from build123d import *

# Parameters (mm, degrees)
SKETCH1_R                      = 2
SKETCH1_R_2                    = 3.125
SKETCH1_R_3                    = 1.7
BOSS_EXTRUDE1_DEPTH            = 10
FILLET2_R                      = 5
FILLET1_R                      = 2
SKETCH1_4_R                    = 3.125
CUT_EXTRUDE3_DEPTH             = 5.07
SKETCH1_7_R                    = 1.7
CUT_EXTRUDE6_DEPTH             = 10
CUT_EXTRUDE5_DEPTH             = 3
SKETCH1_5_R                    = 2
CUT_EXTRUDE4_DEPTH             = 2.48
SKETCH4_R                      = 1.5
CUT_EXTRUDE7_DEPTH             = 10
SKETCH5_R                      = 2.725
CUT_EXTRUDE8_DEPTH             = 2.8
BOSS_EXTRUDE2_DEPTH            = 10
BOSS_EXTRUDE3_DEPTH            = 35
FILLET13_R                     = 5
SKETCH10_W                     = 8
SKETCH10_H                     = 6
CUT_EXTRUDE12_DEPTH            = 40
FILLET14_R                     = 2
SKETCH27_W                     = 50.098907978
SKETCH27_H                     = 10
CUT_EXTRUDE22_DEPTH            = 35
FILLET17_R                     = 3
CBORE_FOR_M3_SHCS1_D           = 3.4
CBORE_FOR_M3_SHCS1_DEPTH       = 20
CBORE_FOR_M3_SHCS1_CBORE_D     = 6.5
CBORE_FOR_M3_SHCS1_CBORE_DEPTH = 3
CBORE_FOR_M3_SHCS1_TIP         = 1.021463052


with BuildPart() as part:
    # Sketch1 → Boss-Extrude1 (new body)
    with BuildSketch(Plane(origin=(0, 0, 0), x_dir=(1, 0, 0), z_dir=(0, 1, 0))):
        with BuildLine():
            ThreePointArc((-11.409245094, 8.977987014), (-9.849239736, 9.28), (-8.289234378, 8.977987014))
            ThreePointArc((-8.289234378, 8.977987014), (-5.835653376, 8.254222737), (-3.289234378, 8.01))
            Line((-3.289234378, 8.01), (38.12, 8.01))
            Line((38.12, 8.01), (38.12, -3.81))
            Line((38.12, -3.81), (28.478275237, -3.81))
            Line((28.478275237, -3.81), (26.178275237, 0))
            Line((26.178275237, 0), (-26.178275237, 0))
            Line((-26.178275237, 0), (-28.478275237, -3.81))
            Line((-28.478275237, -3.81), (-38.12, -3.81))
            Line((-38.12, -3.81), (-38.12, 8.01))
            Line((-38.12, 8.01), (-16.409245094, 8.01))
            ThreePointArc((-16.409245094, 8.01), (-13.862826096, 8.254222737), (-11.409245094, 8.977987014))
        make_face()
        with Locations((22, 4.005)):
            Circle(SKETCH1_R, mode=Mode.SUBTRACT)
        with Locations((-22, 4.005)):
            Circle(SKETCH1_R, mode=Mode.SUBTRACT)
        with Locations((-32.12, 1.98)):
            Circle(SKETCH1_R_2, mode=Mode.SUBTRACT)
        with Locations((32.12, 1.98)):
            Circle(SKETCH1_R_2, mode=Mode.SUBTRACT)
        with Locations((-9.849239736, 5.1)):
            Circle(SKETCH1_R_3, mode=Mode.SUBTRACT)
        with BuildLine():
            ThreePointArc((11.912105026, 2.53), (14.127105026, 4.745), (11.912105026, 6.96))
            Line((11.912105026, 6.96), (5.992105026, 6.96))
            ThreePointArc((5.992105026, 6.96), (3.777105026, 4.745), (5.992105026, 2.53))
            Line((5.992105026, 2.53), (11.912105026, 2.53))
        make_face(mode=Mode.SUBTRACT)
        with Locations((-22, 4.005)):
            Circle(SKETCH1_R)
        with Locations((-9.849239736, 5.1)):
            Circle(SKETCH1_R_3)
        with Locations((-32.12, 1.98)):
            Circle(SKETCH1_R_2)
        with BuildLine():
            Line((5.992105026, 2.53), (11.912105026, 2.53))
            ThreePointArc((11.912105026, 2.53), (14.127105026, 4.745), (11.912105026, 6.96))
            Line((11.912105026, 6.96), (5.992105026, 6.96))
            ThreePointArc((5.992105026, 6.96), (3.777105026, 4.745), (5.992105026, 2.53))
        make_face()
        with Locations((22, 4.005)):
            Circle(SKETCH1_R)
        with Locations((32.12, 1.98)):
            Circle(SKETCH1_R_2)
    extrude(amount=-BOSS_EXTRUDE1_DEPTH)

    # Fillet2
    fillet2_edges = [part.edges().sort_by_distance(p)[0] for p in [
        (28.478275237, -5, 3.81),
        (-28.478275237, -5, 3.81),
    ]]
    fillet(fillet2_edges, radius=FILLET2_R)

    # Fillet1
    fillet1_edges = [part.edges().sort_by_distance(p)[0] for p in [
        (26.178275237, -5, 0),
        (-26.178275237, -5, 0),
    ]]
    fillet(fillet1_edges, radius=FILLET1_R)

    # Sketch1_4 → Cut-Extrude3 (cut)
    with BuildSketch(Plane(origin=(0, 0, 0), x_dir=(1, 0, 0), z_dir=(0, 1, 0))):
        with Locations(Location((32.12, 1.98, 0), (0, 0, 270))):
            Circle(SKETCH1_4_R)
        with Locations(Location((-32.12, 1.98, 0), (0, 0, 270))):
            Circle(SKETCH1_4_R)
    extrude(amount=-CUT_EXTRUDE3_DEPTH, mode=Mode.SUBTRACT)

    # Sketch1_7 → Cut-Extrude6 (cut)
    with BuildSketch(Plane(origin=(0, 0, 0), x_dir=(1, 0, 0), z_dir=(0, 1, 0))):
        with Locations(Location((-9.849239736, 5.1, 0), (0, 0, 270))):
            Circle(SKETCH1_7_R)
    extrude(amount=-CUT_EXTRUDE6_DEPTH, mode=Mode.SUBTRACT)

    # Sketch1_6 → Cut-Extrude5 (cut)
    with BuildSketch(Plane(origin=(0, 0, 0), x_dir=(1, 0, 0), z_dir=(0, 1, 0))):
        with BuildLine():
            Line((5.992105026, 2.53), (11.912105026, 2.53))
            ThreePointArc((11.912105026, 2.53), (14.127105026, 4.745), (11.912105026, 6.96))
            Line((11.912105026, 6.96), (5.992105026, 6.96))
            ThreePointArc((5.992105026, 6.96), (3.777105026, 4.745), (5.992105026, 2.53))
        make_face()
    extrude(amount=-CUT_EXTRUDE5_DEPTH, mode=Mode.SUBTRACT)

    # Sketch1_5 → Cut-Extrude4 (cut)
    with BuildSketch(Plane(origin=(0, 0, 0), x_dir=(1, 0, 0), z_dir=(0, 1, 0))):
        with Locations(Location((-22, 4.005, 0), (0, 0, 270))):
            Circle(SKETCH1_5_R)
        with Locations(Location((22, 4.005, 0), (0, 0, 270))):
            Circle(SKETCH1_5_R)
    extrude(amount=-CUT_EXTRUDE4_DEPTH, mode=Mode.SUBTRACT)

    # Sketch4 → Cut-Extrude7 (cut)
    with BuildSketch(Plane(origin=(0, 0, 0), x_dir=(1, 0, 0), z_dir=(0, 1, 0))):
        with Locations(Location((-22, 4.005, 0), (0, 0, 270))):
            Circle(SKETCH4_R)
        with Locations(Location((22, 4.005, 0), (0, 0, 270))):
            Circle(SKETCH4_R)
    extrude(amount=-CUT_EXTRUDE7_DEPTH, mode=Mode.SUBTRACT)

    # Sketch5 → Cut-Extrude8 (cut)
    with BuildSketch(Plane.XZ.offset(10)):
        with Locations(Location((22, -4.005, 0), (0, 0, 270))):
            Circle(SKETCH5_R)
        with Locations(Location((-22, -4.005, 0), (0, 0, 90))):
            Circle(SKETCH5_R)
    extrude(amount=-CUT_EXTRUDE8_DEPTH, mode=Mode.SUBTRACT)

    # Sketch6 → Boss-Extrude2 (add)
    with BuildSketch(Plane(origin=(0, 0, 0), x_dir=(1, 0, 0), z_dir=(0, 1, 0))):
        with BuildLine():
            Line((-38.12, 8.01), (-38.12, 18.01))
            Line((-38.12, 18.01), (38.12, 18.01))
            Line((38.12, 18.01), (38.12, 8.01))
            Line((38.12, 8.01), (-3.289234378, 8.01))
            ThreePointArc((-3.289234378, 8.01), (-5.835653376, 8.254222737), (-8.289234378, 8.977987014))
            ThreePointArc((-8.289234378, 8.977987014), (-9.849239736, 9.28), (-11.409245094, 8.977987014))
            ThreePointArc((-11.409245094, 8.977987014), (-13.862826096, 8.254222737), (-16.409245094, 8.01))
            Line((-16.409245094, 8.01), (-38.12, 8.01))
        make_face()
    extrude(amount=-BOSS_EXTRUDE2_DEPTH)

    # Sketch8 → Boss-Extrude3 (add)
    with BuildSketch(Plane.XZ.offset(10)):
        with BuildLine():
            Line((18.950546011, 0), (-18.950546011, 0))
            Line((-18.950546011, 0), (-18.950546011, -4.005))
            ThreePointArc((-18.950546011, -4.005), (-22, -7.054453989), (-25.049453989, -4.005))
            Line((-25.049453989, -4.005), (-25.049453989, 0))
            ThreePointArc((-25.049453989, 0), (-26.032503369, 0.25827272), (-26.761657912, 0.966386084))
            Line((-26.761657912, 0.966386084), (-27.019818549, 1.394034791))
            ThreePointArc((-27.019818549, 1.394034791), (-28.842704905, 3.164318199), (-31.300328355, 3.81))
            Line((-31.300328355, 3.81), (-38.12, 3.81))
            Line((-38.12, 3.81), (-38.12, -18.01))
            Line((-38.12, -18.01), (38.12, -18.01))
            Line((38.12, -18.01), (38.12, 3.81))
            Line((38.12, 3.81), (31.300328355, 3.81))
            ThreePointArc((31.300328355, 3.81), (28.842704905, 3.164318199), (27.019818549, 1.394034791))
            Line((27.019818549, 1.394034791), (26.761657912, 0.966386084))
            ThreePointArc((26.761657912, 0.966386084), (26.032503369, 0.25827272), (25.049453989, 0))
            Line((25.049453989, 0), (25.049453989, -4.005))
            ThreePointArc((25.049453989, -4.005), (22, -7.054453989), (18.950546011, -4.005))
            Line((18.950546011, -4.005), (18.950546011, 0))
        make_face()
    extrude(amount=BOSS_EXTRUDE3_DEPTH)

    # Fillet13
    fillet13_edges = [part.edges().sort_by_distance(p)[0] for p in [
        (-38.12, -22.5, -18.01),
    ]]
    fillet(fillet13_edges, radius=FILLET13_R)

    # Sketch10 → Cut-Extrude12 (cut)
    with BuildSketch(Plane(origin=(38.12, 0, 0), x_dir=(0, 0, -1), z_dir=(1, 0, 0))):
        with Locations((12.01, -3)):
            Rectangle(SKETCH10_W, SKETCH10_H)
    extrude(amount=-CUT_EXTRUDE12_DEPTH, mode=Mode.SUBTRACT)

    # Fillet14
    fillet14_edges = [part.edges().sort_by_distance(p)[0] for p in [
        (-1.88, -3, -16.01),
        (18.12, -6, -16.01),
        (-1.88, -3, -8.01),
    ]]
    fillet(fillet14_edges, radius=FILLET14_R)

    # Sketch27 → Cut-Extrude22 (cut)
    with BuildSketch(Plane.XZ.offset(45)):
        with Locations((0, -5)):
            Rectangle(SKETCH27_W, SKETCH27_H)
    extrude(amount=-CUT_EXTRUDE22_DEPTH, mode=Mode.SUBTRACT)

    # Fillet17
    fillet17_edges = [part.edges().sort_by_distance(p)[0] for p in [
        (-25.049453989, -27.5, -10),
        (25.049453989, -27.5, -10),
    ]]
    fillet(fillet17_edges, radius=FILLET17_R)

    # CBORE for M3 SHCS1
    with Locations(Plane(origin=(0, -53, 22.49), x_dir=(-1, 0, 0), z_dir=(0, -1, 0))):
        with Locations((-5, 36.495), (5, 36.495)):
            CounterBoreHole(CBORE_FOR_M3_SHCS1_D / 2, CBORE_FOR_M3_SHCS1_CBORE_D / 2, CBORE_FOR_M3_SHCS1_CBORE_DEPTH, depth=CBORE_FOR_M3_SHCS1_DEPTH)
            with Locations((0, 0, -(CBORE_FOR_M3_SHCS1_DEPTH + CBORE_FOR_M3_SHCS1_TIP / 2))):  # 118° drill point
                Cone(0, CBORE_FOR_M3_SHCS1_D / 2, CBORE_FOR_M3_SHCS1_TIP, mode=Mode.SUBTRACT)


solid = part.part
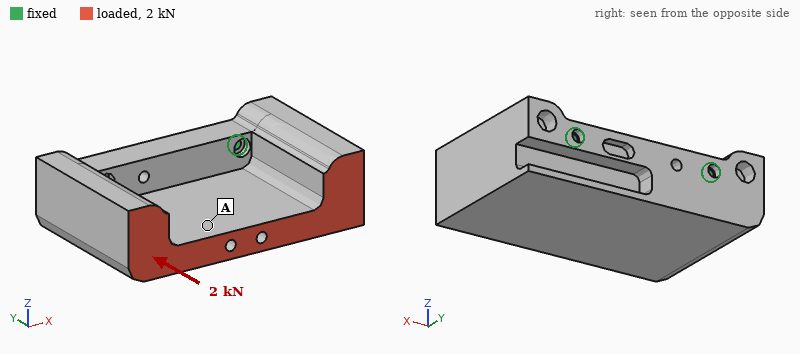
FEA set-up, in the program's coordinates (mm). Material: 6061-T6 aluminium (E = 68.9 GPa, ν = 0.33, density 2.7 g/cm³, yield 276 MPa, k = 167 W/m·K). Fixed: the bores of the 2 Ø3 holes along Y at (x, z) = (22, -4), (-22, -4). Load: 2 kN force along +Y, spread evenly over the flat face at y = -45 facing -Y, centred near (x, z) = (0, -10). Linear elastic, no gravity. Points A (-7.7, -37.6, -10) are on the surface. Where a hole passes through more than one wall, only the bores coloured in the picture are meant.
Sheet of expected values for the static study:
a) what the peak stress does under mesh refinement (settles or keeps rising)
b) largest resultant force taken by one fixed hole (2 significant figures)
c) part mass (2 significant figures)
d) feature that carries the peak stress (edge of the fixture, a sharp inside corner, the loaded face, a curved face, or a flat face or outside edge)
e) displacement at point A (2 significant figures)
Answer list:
keeps rising
1.0 kN
120 g
edge of the fixture
55 µm
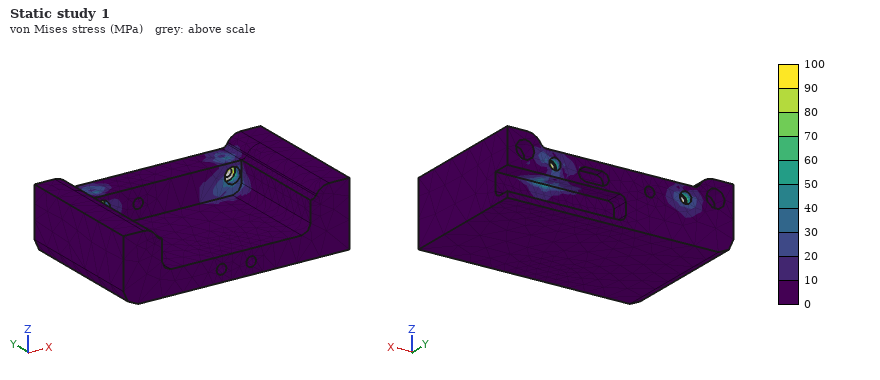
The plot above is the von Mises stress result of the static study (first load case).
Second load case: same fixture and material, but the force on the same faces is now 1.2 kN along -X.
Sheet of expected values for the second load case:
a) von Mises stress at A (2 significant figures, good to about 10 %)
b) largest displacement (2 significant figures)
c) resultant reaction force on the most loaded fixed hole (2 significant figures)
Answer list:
13 MPa
51 µm
1.2 kN
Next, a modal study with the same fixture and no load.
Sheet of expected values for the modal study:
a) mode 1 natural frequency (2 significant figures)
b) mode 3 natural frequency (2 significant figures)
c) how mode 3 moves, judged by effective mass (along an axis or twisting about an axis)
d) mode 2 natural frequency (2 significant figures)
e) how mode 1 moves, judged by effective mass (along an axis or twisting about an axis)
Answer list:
1600 Hz
6600 Hz
along X
3200 Hz
along Z
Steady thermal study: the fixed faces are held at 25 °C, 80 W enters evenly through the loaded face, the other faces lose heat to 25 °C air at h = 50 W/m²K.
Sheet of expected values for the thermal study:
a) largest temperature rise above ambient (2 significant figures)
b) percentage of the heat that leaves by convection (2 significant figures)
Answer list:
32 K
14 %
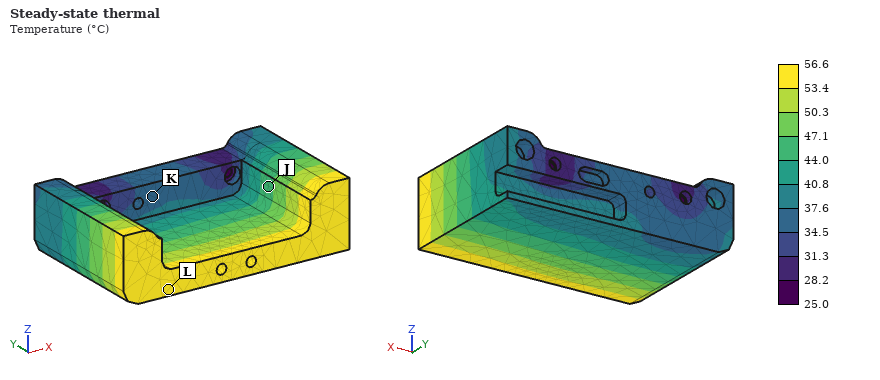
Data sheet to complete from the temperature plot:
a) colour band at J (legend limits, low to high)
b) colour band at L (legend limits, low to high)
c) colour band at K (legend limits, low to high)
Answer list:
44.0 to 47.1 °C
53.4 to 56.6 °C
34.5 to 37.6 °C
